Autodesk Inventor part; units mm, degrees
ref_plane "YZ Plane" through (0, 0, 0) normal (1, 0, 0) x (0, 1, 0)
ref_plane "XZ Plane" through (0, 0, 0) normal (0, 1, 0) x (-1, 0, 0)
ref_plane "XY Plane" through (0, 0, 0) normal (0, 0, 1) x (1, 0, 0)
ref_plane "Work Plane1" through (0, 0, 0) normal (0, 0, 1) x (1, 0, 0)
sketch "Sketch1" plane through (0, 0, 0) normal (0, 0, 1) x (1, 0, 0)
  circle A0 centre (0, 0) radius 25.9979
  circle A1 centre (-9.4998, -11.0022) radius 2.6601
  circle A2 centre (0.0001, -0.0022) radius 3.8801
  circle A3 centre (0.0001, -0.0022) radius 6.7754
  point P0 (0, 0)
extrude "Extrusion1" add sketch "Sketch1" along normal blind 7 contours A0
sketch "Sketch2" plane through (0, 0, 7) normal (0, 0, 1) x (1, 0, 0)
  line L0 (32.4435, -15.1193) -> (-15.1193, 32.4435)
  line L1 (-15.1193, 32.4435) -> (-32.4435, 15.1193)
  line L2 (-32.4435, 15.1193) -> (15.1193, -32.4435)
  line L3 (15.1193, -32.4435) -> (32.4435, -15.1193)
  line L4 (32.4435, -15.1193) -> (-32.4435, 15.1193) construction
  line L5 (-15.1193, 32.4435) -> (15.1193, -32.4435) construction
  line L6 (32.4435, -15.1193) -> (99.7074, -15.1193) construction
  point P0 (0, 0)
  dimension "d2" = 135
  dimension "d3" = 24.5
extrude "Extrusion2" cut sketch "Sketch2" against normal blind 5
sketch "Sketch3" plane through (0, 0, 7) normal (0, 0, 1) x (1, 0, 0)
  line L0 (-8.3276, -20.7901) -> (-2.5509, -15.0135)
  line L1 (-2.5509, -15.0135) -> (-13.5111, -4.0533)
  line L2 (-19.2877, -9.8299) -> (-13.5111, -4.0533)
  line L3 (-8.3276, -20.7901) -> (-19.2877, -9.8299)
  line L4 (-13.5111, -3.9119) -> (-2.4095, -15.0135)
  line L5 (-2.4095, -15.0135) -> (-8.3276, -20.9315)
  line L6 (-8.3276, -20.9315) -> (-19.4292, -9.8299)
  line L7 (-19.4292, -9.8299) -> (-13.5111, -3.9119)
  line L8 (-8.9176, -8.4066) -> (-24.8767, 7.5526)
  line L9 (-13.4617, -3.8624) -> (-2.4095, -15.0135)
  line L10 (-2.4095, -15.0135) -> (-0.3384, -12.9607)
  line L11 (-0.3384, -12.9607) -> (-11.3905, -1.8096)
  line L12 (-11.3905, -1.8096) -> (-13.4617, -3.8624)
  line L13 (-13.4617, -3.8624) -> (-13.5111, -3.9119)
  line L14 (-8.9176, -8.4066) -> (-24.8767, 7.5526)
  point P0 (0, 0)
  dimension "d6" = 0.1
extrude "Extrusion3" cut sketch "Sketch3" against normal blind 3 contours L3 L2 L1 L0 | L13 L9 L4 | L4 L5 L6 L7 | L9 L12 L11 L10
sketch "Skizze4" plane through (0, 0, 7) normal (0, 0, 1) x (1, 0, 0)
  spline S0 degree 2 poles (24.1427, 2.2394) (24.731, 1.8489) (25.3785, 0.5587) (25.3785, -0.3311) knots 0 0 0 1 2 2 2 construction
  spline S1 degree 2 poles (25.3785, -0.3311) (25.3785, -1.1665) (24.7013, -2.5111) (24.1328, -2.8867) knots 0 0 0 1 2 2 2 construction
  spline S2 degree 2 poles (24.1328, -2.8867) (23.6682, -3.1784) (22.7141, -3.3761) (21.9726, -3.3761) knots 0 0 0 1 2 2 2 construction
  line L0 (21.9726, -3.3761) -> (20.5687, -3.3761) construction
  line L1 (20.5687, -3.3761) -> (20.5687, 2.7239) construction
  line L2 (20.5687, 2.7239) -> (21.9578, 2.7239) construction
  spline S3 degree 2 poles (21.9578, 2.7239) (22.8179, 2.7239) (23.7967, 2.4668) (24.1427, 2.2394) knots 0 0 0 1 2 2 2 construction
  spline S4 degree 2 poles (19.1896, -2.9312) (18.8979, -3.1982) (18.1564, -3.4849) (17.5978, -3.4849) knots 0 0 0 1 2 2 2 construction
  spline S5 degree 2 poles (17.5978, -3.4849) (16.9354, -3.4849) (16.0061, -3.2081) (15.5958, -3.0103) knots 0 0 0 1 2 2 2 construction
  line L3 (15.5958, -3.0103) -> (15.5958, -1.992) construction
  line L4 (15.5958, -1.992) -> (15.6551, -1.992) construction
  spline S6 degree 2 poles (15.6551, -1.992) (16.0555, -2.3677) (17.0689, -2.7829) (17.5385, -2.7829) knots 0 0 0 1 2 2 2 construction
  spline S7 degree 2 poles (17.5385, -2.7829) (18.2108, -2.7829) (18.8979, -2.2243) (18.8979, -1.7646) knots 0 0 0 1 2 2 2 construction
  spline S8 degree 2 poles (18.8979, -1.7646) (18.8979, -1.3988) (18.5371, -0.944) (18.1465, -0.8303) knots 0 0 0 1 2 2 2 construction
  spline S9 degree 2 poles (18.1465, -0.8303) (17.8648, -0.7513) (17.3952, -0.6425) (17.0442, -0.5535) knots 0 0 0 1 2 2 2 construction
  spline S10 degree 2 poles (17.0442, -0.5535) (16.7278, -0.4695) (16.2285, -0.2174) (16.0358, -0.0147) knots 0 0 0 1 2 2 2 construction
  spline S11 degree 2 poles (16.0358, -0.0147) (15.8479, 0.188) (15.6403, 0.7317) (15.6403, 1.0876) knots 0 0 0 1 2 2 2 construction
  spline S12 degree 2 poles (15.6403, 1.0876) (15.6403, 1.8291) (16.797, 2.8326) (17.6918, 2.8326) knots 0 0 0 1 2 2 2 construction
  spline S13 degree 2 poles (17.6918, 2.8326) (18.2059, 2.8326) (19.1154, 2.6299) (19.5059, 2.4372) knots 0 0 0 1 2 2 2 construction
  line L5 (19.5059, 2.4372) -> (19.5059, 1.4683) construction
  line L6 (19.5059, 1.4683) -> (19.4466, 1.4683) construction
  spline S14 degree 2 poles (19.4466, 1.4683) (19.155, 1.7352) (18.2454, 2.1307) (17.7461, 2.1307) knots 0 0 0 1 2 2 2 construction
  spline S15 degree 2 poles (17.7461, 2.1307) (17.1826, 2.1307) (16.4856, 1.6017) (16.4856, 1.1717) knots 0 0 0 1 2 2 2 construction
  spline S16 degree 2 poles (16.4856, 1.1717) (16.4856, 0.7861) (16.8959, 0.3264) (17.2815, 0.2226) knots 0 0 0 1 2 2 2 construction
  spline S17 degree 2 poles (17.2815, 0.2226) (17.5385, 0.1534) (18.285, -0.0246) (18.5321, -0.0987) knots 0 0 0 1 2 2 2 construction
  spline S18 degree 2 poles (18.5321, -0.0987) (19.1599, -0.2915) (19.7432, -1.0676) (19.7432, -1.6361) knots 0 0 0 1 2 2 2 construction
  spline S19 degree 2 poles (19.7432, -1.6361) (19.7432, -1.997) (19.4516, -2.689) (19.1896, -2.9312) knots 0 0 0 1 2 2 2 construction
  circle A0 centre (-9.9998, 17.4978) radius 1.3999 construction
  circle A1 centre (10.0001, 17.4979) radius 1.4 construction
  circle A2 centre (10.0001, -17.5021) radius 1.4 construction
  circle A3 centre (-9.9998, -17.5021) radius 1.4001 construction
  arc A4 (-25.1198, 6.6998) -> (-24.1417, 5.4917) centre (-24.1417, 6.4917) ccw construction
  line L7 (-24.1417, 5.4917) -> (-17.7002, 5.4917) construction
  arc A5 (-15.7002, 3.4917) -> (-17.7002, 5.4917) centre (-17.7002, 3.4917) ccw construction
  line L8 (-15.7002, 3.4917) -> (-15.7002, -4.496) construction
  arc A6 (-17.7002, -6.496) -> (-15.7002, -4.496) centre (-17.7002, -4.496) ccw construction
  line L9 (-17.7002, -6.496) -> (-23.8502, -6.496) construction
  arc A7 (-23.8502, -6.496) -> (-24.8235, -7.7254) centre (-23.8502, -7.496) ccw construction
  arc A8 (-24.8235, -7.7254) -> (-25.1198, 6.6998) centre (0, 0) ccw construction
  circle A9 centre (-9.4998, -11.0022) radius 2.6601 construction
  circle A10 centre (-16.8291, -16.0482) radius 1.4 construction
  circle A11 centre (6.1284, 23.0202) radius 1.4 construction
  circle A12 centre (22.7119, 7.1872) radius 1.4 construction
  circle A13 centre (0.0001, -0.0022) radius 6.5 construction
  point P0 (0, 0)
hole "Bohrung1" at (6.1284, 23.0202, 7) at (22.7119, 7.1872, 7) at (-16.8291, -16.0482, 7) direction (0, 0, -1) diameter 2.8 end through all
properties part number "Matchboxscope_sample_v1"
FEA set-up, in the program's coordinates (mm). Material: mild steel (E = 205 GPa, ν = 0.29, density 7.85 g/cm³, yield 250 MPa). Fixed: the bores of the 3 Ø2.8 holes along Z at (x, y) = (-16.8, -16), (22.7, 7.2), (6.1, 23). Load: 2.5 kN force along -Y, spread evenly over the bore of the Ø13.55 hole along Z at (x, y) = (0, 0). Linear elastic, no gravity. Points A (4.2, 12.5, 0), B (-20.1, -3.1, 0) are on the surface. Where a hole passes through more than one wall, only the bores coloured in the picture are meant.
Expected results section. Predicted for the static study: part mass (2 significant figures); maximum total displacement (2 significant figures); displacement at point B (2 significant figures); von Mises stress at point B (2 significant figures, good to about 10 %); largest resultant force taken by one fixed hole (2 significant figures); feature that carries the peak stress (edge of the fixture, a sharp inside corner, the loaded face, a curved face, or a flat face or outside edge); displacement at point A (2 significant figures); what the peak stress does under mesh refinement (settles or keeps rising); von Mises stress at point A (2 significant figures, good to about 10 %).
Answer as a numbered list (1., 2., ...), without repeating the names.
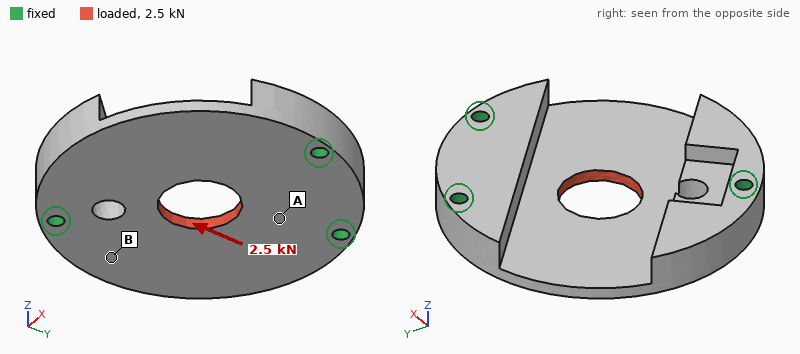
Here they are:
1. 62 g
2. 6.4 µm
3. 2.3 µm
4. 11 MPa
5. 1.0 kN
6. edge of the fixture
7. 1.8 µm
8. keeps rising
9. 37 MPa
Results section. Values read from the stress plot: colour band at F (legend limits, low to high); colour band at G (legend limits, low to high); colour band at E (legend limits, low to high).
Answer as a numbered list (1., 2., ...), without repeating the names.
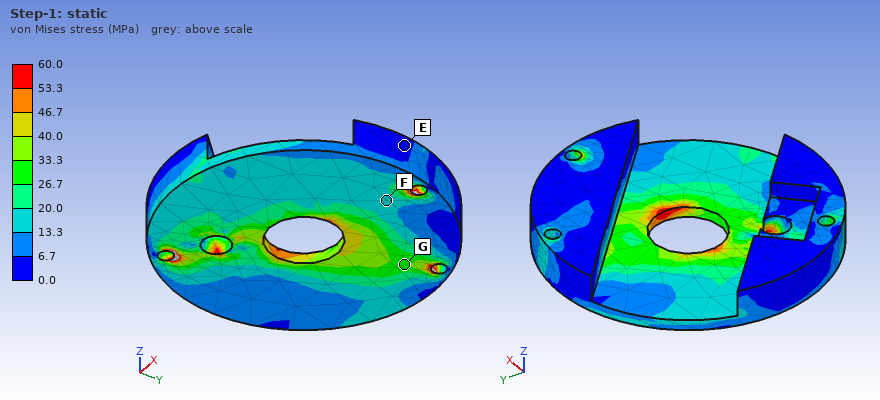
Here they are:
1. 13.3 to 20.0 MPa
2. 26.7 to 33.3 MPa
3. 0.0 to 6.7 MPa
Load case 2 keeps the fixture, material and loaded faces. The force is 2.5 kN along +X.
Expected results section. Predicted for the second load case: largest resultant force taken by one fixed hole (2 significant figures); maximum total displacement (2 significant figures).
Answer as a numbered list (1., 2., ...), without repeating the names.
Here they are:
1. 1.0 kN
2. 5.9 µm
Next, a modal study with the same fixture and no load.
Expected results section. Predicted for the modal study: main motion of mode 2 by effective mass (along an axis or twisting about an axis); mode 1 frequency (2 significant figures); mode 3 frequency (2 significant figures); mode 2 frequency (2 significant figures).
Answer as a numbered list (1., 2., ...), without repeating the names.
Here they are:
1. along Z
2. 7300 Hz
3. 14 kHz
4. 8100 Hz
